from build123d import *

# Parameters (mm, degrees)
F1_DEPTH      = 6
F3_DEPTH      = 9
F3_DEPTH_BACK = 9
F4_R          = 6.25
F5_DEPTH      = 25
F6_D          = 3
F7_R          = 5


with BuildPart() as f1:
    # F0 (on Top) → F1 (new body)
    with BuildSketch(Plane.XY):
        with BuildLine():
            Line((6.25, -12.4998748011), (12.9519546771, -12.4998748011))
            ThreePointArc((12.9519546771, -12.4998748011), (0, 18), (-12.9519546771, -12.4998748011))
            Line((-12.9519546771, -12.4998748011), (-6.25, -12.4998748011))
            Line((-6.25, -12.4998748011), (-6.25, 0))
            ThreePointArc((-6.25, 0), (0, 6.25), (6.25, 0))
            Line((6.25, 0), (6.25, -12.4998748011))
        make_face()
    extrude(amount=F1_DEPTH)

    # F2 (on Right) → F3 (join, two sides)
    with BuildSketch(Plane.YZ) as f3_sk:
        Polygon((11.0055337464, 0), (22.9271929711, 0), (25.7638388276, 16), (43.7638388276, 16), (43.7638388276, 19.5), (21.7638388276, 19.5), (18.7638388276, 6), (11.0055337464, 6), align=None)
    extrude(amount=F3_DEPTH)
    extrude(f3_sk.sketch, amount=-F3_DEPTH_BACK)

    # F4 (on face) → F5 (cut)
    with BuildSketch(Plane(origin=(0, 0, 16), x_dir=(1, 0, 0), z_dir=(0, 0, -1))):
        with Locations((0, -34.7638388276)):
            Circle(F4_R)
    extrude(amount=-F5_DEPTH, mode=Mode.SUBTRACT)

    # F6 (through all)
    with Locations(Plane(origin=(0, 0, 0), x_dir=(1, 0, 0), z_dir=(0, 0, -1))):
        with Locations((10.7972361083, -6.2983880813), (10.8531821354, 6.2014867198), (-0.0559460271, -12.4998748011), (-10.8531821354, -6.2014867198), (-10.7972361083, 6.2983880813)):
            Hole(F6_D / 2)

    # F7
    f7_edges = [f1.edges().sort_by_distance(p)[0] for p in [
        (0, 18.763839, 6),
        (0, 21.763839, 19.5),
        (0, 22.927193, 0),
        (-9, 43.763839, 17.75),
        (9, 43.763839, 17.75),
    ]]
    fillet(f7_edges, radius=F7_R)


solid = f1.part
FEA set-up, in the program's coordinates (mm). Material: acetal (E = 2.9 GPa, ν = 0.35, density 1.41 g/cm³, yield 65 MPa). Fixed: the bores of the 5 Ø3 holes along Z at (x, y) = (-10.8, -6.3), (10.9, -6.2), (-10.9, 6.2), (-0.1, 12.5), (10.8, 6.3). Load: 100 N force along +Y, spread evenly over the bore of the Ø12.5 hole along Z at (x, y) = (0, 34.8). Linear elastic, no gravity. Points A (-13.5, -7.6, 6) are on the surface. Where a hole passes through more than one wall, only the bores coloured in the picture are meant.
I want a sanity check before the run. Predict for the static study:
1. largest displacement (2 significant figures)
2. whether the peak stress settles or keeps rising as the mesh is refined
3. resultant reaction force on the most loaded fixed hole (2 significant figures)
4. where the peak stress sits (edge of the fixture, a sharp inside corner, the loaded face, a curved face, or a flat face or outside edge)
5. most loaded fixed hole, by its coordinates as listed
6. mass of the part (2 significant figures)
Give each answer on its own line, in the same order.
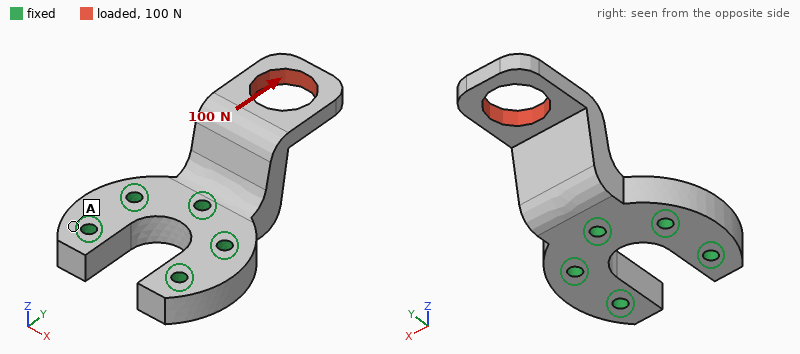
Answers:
0.70 mm
keeps rising
92 N
edge of the fixture
(-0.1, 12.5)
9.1 g
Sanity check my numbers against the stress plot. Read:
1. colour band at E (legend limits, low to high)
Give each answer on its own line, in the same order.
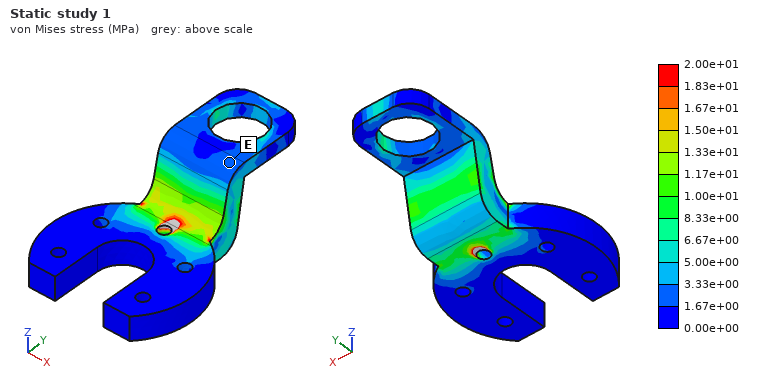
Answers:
1.67e+00 to 3.33e+00 MPa
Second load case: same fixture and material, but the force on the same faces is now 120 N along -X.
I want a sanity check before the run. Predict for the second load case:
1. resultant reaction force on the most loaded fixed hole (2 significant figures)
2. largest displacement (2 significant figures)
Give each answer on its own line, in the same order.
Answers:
140 N
0.71 mm
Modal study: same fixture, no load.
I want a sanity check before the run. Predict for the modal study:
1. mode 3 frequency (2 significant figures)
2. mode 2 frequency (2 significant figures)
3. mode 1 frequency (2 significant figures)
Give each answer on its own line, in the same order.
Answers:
3000 Hz
2400 Hz
1300 Hz
